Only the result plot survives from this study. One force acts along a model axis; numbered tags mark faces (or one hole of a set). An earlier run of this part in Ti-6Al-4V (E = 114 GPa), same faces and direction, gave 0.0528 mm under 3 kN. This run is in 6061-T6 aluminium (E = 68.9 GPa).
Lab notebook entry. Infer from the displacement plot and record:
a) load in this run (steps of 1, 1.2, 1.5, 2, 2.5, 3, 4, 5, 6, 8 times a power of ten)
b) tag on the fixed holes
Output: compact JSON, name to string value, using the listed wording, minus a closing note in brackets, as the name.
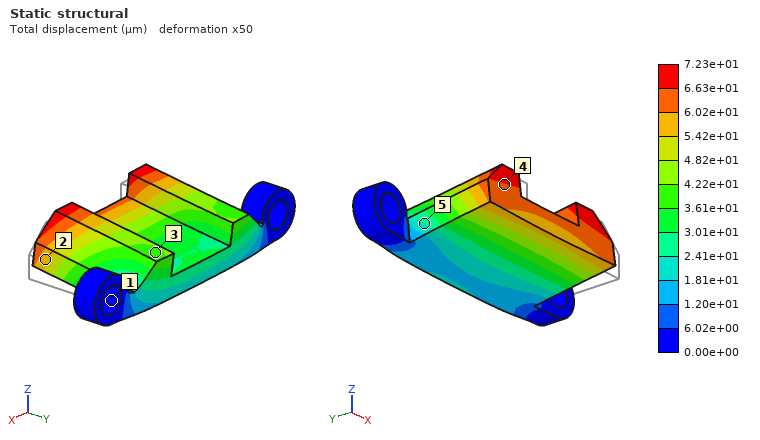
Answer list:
{"load in this run": "2.5 kN", "tag on the fixed holes": "1"}
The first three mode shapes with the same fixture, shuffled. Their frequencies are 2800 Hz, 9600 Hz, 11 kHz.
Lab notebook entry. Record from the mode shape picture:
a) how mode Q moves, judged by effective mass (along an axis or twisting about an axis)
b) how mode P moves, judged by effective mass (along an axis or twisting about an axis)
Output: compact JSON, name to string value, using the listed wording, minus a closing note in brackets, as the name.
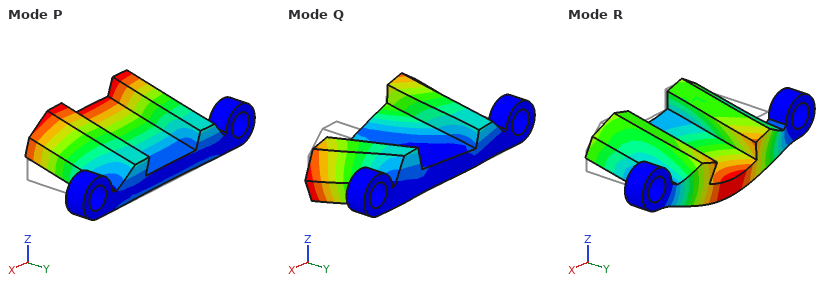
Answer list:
{"how mode Q moves, judged by effective mass": "twisting about Y", "how mode P moves, judged by effective mass": "along Z"}
